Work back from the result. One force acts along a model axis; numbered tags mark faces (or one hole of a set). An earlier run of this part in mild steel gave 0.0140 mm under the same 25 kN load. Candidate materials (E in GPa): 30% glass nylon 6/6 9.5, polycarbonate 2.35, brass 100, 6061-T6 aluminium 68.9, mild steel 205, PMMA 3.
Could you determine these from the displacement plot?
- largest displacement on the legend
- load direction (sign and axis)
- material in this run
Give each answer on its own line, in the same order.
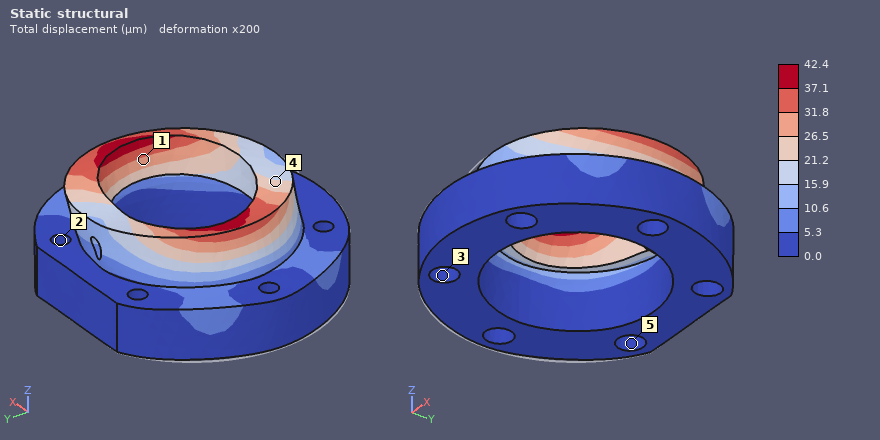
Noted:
42.4 µm
+X
6061-T6 aluminium
